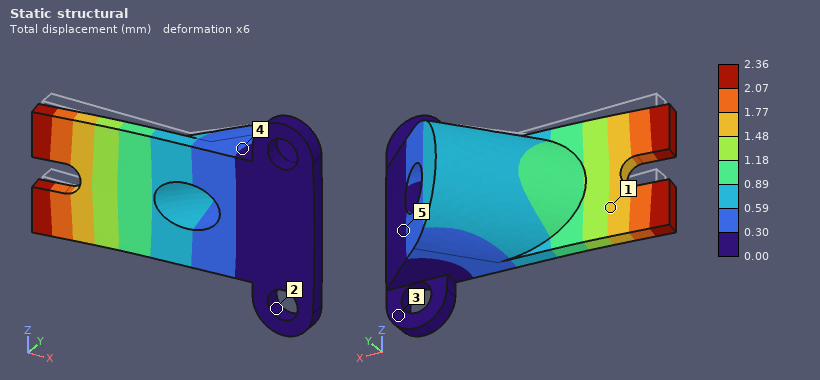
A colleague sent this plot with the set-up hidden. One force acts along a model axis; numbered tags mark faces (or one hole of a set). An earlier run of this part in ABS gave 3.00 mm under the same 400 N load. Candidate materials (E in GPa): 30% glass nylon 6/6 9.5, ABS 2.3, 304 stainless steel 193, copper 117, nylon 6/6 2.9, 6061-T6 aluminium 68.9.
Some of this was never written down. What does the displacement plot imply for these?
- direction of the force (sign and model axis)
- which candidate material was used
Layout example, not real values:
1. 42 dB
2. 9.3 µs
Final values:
1. -Y
2. nylon 6/6
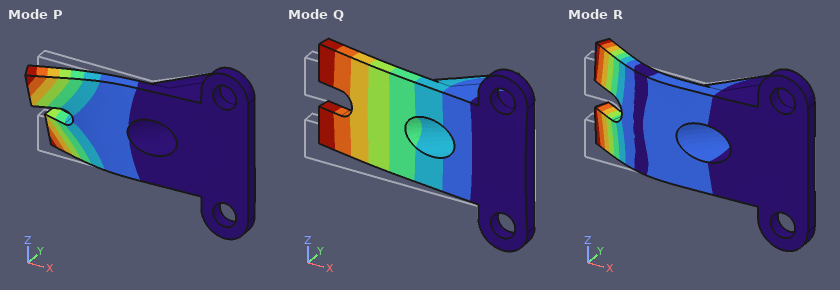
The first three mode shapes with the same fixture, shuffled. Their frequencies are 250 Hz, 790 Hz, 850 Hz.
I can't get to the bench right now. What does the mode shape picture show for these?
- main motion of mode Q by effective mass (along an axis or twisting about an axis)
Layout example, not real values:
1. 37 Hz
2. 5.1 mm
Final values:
1. along Y
